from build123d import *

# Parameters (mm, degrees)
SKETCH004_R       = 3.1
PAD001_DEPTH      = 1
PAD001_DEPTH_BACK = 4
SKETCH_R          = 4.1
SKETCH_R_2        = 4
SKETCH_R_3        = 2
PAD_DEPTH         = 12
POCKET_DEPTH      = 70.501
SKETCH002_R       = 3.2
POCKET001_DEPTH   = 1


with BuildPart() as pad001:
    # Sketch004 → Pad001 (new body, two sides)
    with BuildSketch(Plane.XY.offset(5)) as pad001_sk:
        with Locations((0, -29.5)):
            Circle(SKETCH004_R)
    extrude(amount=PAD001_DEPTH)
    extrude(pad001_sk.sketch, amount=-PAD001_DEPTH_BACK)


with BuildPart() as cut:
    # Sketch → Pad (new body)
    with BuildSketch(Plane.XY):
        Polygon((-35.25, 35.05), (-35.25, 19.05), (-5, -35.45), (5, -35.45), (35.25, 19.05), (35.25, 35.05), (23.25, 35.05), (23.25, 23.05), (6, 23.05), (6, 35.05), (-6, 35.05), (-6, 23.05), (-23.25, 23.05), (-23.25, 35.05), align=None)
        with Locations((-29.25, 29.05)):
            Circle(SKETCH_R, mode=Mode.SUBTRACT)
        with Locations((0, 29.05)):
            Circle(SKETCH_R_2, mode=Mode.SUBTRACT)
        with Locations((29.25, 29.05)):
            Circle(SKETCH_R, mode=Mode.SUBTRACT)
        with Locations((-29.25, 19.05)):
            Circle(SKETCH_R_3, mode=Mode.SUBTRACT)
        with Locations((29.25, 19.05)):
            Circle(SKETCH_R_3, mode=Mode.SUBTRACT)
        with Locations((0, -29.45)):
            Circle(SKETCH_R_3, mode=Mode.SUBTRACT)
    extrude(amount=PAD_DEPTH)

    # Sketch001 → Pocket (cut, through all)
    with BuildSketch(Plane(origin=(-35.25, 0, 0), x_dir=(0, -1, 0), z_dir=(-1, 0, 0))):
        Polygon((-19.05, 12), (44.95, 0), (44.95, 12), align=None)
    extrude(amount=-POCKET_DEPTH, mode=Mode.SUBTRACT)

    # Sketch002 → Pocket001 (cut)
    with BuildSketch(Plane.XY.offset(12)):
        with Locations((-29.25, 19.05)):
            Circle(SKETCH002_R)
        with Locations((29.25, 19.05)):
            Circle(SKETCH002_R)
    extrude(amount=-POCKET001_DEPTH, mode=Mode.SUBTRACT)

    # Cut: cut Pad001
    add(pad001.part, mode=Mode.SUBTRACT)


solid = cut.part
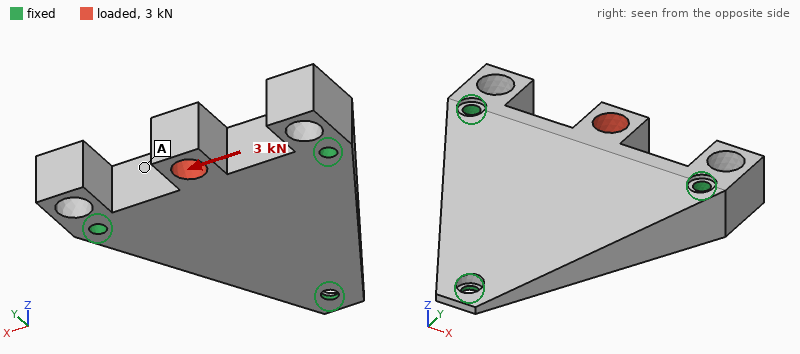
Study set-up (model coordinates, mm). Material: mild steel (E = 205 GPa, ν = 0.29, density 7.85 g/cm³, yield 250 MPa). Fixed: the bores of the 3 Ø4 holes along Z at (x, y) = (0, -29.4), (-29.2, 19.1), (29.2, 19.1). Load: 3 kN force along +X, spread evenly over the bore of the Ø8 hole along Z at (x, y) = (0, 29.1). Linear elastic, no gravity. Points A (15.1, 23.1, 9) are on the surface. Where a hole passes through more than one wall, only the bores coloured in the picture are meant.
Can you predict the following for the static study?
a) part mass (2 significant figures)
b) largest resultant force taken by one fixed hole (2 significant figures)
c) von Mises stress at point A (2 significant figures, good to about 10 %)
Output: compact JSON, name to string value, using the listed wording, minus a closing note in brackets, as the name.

{"part mass": "190 g", "largest resultant force taken by one fixed hole": "1.6 kN", "von Mises stress at point A": "20 MPa"}
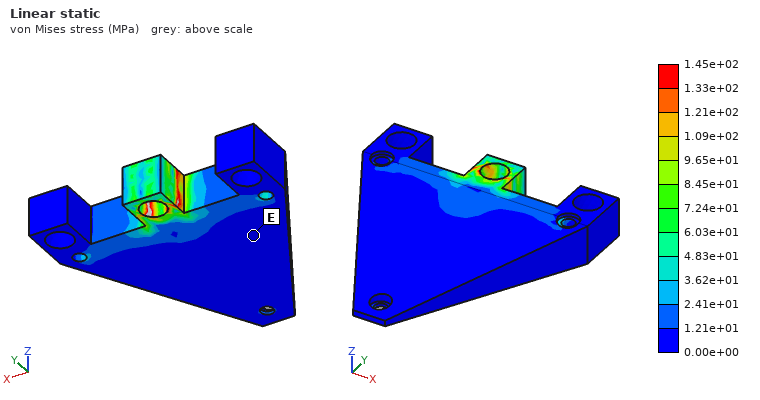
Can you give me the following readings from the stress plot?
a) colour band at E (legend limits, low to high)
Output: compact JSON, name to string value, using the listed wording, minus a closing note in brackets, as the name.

{"colour band at E": "0.00e+00 to 1.21e+01 MPa"}
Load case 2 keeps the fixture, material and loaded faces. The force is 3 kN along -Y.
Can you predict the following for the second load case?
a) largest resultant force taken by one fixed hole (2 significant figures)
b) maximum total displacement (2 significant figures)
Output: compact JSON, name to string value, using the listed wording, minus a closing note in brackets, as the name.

{"largest resultant force taken by one fixed hole": "1.3 kN", "maximum total displacement": "7.2 µm"}
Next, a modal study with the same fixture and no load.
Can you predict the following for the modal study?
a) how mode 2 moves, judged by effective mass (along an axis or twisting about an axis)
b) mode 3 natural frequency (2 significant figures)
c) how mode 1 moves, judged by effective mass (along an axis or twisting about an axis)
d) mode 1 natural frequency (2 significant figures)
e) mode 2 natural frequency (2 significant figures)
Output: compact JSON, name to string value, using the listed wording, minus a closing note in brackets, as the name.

{"how mode 2 moves, judged by effective mass": "along Z", "mode 3 natural frequency": "14 kHz", "how mode 1 moves, judged by effective mass": "along Z", "mode 1 natural frequency": "8100 Hz", "mode 2 natural frequency": "11 kHz"}
